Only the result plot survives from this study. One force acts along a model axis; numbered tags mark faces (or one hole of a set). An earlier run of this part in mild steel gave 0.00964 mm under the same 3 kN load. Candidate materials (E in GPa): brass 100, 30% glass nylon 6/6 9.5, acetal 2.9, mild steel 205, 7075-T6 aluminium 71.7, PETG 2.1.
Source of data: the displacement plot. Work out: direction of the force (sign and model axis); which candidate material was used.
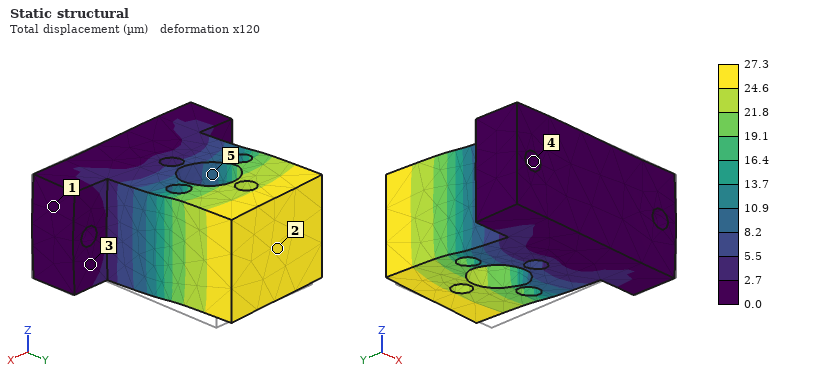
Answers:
-X
7075-T6 aluminium
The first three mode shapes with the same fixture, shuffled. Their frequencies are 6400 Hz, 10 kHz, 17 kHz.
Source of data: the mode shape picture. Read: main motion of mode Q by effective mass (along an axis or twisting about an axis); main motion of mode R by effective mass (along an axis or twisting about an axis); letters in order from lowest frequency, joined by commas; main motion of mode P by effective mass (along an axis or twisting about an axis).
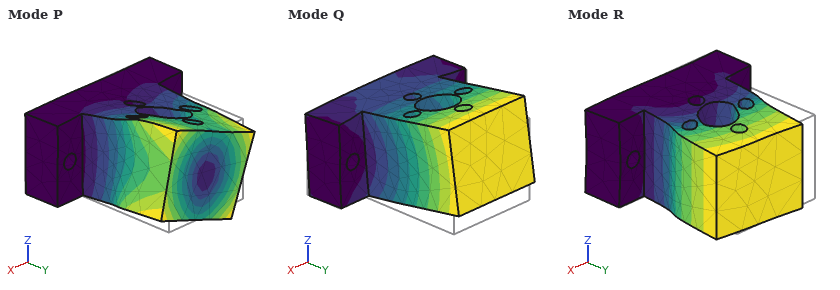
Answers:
along Z
along X
Q, R, P
twisting about Y
